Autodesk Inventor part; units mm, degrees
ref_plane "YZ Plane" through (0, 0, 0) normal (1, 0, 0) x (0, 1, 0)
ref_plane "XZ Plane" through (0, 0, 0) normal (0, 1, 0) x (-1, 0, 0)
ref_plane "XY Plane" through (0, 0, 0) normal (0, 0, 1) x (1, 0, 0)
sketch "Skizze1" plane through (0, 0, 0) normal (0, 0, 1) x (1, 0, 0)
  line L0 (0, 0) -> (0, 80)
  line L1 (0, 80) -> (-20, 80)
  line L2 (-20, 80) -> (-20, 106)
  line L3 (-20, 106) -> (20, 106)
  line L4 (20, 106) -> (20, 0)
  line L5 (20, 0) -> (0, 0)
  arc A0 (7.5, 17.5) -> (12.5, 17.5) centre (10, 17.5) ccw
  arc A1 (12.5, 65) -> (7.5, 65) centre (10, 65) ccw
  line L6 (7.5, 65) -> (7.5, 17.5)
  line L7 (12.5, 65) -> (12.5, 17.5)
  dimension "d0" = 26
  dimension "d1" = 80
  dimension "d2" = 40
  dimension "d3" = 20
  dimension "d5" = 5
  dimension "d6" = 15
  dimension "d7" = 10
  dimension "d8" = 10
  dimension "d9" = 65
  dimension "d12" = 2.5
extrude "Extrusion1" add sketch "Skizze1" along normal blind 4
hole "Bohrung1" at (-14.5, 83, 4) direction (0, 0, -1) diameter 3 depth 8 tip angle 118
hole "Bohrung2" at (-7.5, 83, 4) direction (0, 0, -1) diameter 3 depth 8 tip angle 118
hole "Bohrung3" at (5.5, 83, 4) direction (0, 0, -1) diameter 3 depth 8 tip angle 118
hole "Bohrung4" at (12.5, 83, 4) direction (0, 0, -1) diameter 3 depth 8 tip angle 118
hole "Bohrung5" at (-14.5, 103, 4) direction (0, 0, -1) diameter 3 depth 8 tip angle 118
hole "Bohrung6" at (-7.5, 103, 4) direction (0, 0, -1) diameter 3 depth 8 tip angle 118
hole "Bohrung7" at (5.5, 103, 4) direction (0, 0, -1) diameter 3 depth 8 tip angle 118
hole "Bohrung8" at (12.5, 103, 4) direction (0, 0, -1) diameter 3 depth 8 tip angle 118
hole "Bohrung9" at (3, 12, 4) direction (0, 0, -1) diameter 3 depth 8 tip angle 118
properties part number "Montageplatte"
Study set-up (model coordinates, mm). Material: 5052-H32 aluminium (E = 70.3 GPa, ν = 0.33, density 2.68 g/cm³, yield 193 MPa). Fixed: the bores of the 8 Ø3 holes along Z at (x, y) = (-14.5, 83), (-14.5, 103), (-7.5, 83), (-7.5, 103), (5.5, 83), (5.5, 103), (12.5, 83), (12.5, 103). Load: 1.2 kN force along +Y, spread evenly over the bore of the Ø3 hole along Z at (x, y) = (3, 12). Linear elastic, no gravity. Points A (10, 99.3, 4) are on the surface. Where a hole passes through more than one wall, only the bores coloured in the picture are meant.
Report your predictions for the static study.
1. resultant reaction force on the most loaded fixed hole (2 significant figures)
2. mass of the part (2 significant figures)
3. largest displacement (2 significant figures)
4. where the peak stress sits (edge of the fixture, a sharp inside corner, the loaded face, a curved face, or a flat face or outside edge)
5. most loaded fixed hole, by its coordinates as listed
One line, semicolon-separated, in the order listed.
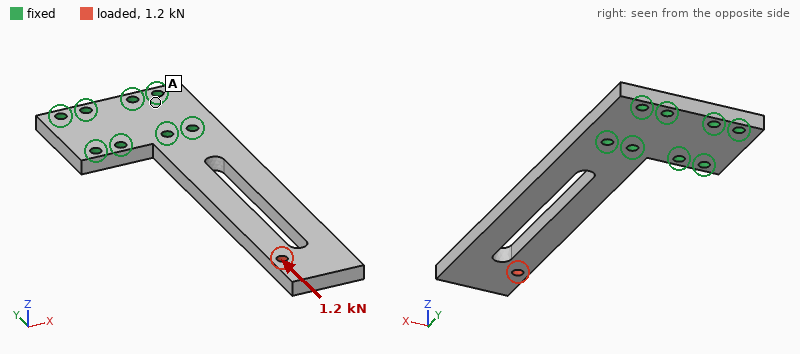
940 N; 25 g; 0.17 mm; the loaded face; (5.5, 83)
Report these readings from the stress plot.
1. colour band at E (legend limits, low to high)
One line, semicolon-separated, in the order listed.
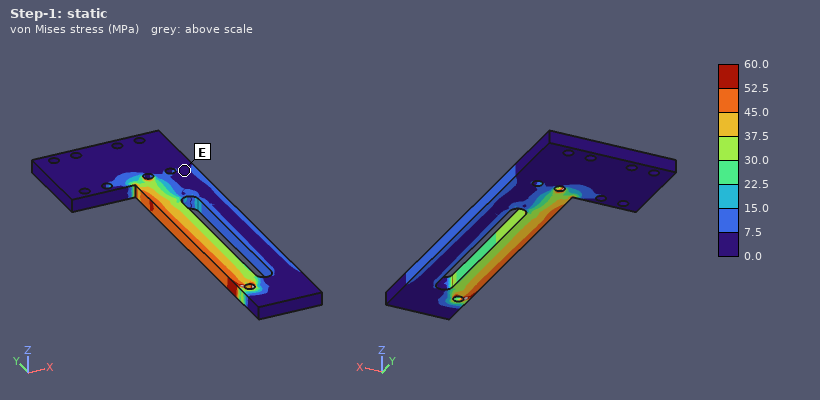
0.0 to 7.5 MPa
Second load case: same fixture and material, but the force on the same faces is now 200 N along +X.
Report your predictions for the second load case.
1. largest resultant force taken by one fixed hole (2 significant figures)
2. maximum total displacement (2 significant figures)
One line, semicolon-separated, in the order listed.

920 N; 0.32 mm
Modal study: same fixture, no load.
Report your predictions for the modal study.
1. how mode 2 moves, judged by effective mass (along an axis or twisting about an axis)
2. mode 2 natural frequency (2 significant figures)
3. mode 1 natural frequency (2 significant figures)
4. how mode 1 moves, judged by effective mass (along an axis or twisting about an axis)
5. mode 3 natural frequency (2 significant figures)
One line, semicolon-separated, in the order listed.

along X; 1700 Hz; 480 Hz; along Z; 2900 Hz
